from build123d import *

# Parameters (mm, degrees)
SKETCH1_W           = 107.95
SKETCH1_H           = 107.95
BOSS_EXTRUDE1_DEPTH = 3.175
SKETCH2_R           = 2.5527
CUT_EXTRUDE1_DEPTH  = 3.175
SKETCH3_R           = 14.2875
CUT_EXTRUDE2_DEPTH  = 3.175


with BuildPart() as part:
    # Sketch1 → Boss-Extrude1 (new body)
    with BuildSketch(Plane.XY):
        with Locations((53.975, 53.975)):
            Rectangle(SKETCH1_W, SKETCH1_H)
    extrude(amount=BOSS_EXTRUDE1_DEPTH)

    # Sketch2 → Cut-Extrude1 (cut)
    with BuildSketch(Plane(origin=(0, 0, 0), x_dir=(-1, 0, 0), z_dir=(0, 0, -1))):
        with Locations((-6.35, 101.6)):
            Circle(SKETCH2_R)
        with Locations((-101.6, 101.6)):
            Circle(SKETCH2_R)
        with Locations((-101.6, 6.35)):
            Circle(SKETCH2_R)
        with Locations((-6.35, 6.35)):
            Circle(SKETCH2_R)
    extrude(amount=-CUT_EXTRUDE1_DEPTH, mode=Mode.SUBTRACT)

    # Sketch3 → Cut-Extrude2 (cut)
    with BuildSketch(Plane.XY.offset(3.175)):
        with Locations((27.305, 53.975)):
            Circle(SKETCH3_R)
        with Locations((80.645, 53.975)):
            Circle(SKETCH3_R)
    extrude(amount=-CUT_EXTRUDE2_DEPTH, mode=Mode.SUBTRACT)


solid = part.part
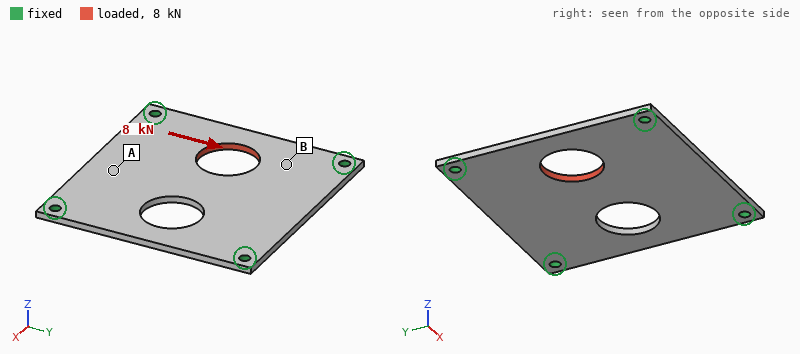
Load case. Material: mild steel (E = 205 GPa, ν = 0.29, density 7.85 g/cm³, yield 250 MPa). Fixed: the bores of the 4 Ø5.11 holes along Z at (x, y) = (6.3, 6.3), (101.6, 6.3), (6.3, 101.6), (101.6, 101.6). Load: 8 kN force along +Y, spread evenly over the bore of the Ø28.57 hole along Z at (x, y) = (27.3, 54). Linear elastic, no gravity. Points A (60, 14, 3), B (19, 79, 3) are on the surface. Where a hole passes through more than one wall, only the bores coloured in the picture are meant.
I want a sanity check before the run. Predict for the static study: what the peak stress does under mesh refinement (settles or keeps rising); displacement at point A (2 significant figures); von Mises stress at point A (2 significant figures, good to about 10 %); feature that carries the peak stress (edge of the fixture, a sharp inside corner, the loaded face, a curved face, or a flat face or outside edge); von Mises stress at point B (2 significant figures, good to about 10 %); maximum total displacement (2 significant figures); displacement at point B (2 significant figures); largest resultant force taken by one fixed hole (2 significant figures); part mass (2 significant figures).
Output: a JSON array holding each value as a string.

["keeps rising", "7.6 µm", "11 MPa", "edge of the fixture", "32 MPa", "11 µm", "7.2 µm", "3.0 kN", "260 g"]
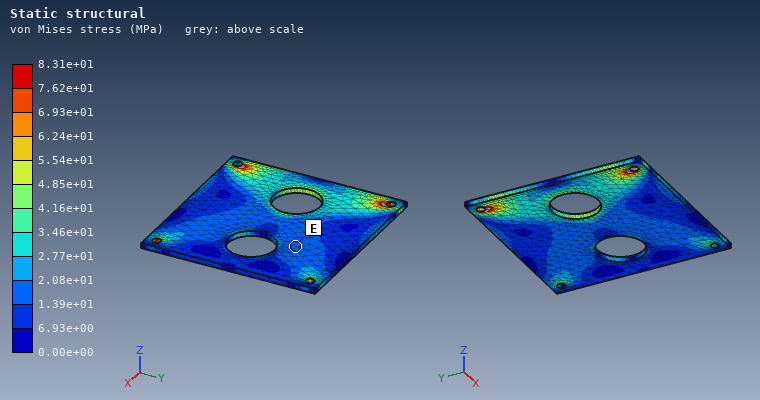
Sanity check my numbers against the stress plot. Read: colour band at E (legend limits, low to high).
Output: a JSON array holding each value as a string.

["1.39e+01 to 2.08e+01 MPa"]
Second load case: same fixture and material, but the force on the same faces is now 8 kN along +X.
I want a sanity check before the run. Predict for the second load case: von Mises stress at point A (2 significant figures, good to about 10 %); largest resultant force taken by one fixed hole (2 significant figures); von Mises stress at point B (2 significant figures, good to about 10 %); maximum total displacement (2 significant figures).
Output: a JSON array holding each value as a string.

["17 MPa", "2.3 kN", "30 MPa", "20 µm"]
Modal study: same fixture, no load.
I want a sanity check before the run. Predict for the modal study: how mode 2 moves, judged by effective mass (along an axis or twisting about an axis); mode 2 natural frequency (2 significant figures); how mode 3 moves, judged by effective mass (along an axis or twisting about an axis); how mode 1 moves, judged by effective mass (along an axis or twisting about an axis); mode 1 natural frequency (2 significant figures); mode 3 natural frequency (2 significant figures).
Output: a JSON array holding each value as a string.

["twisting about X", "2000 Hz", "twisting about Y", "along Z", "1200 Hz", "2200 Hz"]
